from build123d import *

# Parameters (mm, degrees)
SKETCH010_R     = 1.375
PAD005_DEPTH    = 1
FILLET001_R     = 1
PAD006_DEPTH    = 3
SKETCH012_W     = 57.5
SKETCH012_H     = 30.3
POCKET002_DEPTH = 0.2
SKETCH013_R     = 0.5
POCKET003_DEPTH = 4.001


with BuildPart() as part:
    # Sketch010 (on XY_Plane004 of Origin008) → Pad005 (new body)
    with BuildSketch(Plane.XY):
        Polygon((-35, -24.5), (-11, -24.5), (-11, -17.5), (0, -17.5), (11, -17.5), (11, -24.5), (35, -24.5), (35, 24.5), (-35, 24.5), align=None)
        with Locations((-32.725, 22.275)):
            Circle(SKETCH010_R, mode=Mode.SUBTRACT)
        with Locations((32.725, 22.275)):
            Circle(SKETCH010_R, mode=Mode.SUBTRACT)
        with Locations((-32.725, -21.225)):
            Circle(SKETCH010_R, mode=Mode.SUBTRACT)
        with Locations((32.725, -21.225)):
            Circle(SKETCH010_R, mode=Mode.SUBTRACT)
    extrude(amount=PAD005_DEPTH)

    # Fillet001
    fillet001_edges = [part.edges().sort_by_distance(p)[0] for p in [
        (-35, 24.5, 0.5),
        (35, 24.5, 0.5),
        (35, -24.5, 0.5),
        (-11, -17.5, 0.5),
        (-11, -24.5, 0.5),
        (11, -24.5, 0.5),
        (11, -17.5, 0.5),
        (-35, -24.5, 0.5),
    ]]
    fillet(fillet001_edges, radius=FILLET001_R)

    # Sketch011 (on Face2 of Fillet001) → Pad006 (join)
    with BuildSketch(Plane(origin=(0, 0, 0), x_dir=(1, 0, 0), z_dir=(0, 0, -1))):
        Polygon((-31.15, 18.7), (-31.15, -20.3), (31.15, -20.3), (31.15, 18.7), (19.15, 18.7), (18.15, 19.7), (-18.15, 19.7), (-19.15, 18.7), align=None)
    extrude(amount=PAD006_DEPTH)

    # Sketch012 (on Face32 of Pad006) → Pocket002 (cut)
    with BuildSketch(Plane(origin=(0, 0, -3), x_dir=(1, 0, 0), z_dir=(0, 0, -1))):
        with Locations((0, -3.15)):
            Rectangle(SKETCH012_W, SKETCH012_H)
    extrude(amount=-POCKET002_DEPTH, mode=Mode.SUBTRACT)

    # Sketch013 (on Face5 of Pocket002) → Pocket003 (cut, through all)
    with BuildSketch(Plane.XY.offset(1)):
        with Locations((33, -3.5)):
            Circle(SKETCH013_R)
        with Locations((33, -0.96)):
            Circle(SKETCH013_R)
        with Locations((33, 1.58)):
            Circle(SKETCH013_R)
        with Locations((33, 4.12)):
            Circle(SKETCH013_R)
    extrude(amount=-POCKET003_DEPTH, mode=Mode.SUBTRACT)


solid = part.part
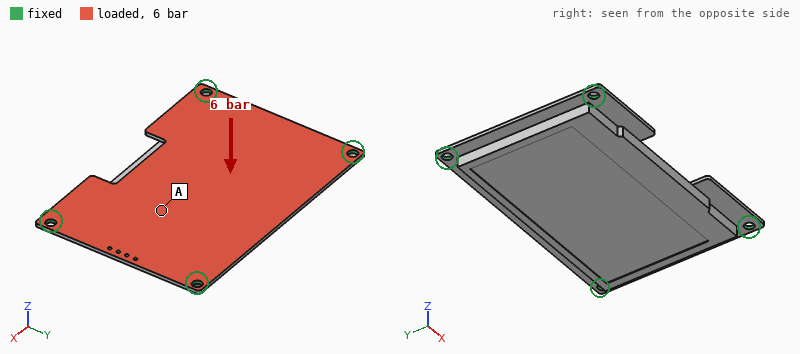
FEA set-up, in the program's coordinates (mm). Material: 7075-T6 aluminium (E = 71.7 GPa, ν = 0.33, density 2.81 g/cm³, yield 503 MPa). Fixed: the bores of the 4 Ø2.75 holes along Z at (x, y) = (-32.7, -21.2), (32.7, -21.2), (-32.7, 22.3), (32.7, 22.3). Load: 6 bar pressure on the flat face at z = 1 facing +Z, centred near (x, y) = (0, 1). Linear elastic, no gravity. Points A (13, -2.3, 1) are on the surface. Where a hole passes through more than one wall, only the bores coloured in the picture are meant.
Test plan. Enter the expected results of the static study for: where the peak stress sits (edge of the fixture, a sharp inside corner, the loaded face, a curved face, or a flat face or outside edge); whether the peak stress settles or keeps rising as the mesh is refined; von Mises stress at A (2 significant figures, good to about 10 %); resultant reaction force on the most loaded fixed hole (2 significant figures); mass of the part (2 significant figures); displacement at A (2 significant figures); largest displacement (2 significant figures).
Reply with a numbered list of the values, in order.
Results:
1. edge of the fixture
2. keeps rising
3. 51 MPa
4. 1.3 kN
5. 29 g
6. 0.27 mm
7. 0.36 mm
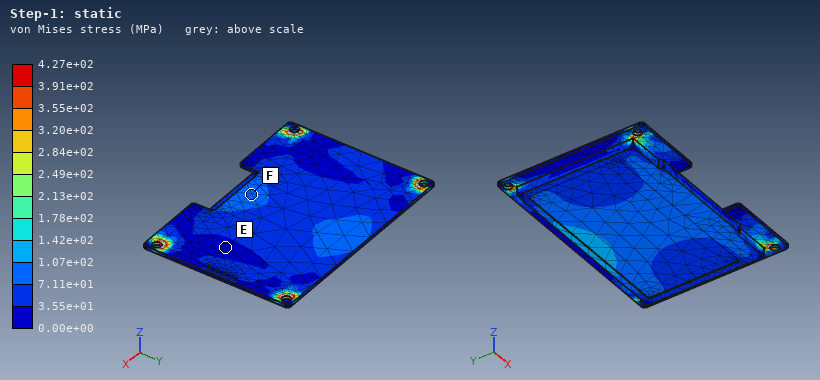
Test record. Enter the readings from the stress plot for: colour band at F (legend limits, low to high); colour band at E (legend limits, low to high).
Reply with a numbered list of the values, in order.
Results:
1. 7.11e+01 to 1.07e+02 MPa
2. 0.00e+00 to 3.55e+01 MPa
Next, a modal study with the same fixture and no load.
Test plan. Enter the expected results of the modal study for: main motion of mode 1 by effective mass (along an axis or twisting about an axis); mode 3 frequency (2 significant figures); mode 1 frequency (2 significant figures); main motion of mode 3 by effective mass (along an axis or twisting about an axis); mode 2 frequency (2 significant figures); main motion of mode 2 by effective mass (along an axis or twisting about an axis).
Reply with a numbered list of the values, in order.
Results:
1. along Z
2. 5800 Hz
3. 2500 Hz
4. twisting about Y
5. 4700 Hz
6. twisting about X
